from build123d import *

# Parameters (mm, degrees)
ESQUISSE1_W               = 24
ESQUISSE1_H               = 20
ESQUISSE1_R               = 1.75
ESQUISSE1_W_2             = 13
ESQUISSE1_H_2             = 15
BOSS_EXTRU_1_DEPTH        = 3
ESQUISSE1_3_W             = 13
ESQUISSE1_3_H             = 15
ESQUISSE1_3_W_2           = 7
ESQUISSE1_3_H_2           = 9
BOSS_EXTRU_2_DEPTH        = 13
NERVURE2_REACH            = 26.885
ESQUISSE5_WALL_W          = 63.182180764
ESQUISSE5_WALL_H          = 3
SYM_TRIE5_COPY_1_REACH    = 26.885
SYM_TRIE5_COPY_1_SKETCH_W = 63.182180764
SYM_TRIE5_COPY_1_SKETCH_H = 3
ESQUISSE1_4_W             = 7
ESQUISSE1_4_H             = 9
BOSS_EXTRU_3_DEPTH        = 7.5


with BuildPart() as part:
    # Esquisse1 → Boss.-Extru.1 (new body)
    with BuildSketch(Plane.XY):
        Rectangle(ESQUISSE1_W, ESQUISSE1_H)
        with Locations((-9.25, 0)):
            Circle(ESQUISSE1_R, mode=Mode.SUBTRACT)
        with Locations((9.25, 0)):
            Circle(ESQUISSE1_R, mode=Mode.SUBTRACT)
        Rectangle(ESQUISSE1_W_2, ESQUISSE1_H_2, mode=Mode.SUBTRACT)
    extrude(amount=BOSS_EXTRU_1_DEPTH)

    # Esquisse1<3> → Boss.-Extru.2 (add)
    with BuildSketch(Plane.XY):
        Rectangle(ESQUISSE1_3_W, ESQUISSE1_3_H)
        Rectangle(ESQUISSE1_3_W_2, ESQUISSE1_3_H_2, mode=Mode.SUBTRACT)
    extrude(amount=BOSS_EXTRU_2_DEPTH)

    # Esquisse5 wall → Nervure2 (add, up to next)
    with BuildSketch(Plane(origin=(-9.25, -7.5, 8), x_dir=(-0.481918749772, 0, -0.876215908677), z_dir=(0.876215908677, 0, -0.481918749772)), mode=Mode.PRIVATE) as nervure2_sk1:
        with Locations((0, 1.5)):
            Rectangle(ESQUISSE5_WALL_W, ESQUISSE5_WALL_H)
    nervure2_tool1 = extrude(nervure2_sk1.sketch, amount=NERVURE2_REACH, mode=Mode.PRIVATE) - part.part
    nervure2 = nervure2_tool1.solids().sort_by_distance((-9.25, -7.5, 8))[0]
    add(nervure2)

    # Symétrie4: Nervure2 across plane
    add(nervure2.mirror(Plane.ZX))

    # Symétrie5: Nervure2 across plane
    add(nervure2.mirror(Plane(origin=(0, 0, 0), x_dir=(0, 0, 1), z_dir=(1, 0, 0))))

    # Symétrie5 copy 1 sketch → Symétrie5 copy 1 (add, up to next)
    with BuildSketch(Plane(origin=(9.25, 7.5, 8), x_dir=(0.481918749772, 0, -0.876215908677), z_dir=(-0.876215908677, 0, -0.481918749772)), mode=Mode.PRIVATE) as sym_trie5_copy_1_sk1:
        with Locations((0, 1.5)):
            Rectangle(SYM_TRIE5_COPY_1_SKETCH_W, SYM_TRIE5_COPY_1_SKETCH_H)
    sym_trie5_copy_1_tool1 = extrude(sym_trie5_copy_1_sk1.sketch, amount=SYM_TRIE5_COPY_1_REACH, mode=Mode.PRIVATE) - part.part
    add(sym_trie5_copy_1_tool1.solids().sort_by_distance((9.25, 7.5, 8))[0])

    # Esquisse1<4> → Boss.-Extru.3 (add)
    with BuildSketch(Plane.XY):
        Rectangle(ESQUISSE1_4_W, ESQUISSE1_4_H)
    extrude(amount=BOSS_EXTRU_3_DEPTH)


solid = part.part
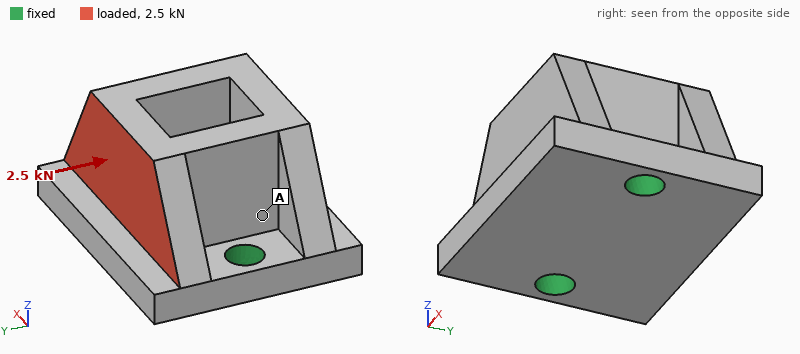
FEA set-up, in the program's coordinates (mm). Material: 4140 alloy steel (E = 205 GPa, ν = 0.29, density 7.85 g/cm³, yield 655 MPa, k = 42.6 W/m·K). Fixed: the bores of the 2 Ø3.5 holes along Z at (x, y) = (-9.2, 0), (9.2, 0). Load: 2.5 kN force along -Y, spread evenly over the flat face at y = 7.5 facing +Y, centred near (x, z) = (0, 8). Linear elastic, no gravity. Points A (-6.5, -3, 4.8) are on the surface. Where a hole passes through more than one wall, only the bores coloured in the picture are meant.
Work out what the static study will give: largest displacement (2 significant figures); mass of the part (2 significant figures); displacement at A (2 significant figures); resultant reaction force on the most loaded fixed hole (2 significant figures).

27 µm
26 g
8.4 µm
1.3 kN
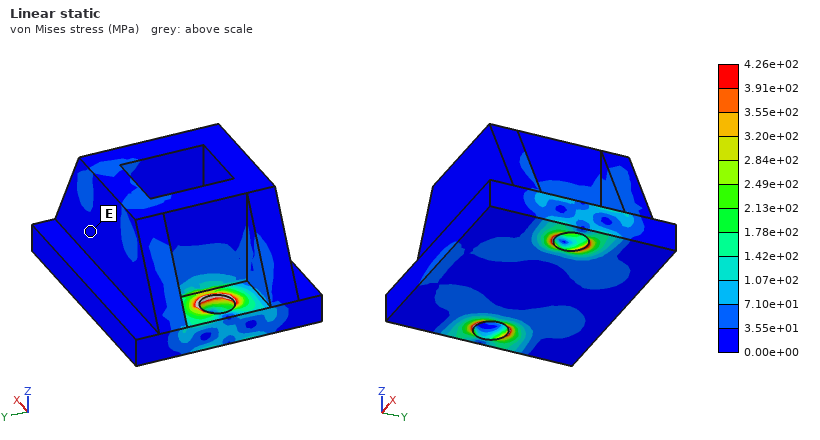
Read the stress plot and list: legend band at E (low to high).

0.00e+00 to 3.55e+01 MPa
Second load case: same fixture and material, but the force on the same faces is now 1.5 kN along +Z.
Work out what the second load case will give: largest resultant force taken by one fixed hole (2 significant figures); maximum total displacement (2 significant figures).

790 N
19 µm
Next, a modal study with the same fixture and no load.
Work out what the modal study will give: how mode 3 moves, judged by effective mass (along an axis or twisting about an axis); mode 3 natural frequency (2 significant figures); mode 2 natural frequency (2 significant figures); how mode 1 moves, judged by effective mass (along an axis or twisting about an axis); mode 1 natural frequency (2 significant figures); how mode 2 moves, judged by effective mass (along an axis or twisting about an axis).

along X
33 kHz
31 kHz
along Y
13 kHz
along Z
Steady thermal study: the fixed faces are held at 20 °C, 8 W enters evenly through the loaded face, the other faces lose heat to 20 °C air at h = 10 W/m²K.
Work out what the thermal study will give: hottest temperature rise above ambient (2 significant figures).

20 K
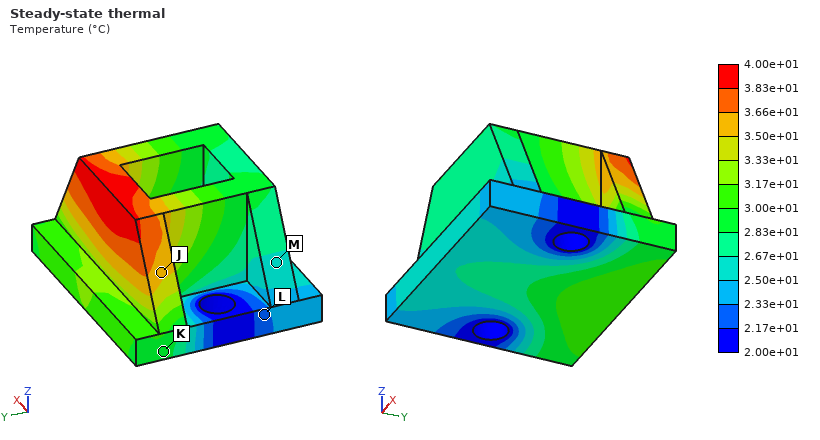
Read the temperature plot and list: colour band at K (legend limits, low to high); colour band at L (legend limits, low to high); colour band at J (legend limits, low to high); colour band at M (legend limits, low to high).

2.83e+01 to 3.00e+01 °C
2.17e+01 to 2.33e+01 °C
3.50e+01 to 3.66e+01 °C
2.50e+01 to 2.67e+01 °C
